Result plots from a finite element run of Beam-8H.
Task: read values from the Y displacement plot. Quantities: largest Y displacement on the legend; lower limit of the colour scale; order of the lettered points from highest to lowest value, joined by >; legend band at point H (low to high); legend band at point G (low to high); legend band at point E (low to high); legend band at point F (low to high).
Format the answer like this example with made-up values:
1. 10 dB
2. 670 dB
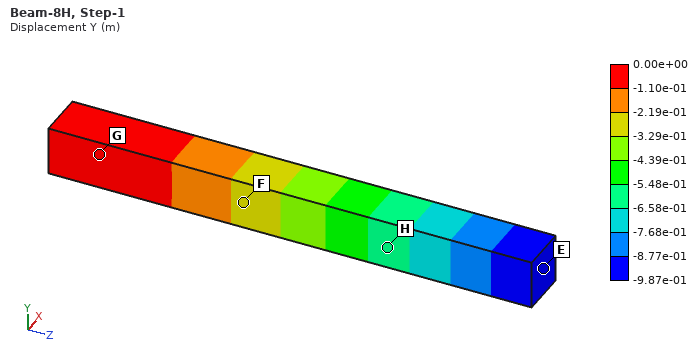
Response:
1. 0.00e+00 m
2. -9.87e-01 m
3. G > F > H > E
4. -6.58e-01 to -5.48e-01 m
5. -1.10e-01 to 0.00e+00 m
6. -9.87e-01 to -8.77e-01 m
7. -3.29e-01 to -2.19e-01 m
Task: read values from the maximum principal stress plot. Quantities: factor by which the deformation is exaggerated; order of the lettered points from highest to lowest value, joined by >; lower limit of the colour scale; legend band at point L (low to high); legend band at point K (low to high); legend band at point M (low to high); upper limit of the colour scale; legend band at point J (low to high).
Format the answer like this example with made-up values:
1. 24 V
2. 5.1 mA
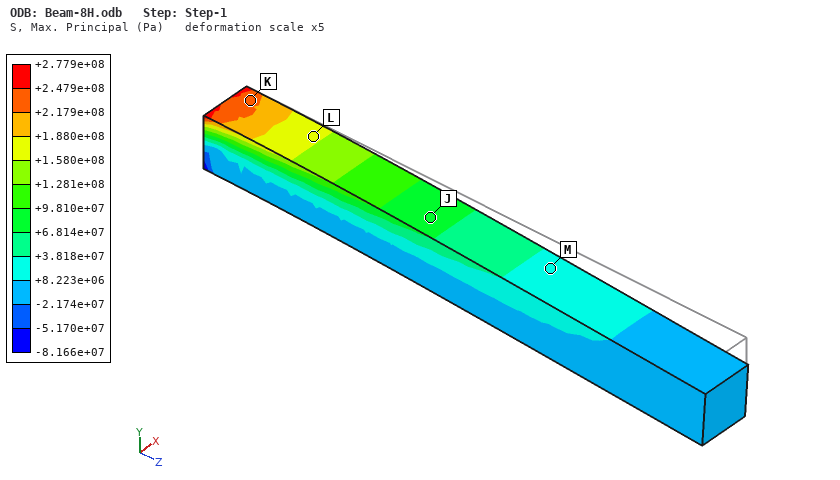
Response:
1. 5
2. K > L > J > M
3. -8.166e+07 Pa
4. +1.580e+08 to +1.880e+08 Pa
5. +2.179e+08 to +2.479e+08 Pa
6. +8.223e+06 to +3.818e+07 Pa
7. +2.779e+08 Pa
8. +6.814e+07 to +9.810e+07 Pa
